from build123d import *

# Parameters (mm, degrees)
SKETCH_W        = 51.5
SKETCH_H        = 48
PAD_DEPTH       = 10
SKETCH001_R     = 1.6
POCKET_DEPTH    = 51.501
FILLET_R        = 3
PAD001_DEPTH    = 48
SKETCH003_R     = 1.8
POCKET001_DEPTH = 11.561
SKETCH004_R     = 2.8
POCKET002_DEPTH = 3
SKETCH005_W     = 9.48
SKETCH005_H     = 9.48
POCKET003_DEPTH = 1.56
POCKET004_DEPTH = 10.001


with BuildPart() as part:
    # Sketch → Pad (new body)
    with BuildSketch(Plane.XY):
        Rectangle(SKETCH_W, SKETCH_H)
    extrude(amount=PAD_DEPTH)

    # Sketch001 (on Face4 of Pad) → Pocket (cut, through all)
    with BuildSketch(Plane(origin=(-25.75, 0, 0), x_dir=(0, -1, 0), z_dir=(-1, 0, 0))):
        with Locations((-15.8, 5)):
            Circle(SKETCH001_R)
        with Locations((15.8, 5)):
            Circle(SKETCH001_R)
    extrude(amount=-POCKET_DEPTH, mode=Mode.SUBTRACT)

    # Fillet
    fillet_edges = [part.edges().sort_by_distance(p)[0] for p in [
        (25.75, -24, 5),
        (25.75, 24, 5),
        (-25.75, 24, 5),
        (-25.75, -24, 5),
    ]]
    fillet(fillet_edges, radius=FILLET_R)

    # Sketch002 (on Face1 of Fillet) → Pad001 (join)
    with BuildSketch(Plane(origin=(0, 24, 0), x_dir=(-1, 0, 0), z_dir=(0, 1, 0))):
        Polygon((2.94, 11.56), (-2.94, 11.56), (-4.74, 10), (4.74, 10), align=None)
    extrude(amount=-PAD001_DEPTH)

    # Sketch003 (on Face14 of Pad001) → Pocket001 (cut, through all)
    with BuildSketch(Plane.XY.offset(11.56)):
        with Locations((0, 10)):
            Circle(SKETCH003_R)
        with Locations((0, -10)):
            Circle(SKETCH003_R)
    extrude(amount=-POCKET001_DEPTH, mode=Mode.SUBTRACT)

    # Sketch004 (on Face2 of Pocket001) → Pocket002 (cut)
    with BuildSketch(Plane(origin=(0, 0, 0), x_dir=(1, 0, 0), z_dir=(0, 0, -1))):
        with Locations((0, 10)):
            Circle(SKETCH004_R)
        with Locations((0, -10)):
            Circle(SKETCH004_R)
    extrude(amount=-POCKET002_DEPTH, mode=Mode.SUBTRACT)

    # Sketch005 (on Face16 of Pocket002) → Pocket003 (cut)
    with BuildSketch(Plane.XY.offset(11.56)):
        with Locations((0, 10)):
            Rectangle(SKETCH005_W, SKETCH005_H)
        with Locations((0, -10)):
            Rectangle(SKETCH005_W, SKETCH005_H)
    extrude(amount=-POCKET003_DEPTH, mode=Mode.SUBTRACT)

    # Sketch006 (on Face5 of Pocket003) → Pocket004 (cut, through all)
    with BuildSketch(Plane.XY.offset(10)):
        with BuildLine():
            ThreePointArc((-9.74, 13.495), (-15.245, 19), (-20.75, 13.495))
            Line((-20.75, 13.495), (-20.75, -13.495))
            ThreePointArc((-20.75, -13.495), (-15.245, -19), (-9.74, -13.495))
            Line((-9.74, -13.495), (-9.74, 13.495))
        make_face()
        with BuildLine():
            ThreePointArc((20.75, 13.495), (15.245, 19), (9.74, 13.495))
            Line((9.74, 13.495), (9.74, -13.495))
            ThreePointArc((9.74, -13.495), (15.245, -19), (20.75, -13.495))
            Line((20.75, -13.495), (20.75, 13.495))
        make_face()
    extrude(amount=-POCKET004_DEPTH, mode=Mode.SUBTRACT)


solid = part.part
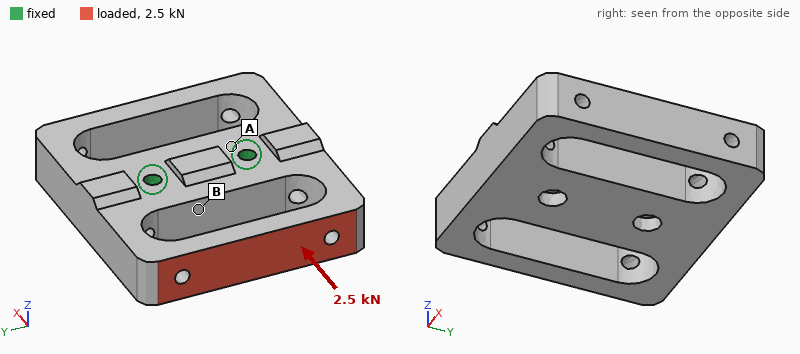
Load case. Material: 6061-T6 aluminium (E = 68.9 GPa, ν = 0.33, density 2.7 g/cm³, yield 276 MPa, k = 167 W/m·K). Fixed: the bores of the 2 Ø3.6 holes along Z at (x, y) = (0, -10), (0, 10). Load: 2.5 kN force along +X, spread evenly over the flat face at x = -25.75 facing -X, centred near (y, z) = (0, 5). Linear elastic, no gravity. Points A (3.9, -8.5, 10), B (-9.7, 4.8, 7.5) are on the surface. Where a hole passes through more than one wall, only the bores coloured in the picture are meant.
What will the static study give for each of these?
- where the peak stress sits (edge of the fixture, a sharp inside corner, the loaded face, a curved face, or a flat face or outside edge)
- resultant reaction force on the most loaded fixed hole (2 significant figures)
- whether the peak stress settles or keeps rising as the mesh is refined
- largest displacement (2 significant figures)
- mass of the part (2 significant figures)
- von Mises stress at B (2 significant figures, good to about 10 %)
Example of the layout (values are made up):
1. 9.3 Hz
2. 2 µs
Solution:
1. a sharp inside corner
2. 1.3 kN
3. keeps rising
4. 0.11 mm
5. 44 g
6. 27 MPa
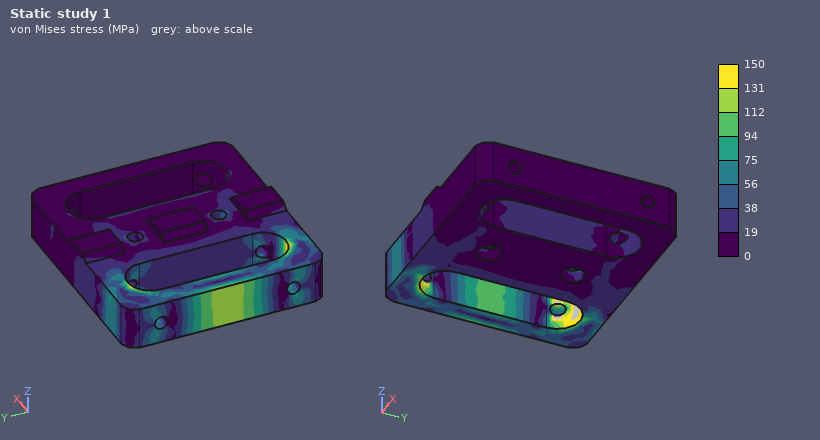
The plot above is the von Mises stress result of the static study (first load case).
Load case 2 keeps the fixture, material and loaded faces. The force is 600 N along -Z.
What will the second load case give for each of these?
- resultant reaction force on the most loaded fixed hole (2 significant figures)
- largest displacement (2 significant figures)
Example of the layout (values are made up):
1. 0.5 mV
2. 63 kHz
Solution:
1. 310 N
2. 83 µm
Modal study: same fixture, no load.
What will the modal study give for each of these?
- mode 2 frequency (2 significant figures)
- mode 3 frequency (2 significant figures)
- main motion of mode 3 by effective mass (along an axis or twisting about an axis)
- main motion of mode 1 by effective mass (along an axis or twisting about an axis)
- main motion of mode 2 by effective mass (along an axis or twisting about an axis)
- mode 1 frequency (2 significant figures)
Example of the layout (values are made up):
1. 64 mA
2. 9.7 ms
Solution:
1. 7300 Hz
2. 7900 Hz
3. twisting about Z
4. twisting about Y
5. along Z
6. 5200 Hz
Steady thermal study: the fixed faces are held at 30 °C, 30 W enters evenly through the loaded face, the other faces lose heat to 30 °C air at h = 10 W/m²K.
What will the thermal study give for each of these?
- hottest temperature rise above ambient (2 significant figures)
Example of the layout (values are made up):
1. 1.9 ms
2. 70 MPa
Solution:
1. 49 K
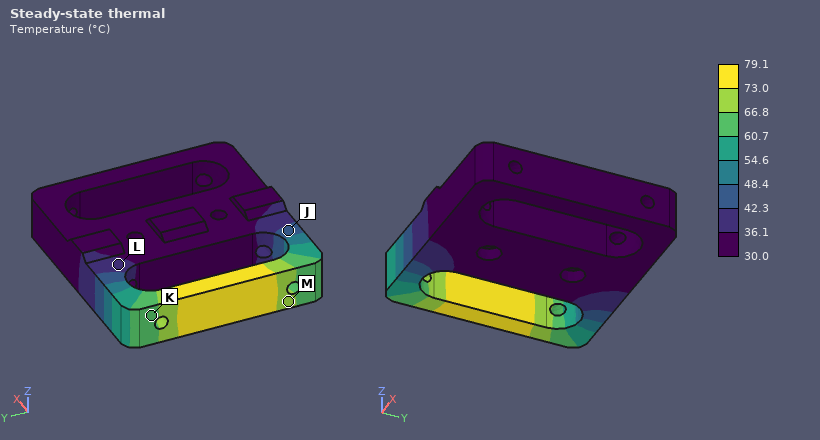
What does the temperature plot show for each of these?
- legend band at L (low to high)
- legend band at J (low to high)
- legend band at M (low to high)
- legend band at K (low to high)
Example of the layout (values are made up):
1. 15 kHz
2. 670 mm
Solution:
1. 36.1 to 42.3 °C
2. 42.3 to 48.4 °C
3. 66.8 to 73.0 °C
4. 60.7 to 66.8 °C
